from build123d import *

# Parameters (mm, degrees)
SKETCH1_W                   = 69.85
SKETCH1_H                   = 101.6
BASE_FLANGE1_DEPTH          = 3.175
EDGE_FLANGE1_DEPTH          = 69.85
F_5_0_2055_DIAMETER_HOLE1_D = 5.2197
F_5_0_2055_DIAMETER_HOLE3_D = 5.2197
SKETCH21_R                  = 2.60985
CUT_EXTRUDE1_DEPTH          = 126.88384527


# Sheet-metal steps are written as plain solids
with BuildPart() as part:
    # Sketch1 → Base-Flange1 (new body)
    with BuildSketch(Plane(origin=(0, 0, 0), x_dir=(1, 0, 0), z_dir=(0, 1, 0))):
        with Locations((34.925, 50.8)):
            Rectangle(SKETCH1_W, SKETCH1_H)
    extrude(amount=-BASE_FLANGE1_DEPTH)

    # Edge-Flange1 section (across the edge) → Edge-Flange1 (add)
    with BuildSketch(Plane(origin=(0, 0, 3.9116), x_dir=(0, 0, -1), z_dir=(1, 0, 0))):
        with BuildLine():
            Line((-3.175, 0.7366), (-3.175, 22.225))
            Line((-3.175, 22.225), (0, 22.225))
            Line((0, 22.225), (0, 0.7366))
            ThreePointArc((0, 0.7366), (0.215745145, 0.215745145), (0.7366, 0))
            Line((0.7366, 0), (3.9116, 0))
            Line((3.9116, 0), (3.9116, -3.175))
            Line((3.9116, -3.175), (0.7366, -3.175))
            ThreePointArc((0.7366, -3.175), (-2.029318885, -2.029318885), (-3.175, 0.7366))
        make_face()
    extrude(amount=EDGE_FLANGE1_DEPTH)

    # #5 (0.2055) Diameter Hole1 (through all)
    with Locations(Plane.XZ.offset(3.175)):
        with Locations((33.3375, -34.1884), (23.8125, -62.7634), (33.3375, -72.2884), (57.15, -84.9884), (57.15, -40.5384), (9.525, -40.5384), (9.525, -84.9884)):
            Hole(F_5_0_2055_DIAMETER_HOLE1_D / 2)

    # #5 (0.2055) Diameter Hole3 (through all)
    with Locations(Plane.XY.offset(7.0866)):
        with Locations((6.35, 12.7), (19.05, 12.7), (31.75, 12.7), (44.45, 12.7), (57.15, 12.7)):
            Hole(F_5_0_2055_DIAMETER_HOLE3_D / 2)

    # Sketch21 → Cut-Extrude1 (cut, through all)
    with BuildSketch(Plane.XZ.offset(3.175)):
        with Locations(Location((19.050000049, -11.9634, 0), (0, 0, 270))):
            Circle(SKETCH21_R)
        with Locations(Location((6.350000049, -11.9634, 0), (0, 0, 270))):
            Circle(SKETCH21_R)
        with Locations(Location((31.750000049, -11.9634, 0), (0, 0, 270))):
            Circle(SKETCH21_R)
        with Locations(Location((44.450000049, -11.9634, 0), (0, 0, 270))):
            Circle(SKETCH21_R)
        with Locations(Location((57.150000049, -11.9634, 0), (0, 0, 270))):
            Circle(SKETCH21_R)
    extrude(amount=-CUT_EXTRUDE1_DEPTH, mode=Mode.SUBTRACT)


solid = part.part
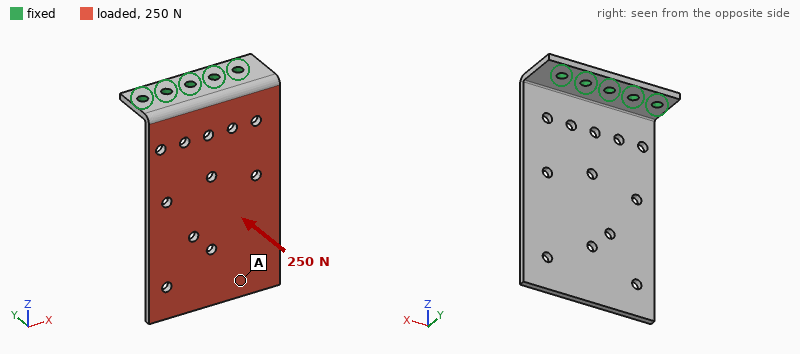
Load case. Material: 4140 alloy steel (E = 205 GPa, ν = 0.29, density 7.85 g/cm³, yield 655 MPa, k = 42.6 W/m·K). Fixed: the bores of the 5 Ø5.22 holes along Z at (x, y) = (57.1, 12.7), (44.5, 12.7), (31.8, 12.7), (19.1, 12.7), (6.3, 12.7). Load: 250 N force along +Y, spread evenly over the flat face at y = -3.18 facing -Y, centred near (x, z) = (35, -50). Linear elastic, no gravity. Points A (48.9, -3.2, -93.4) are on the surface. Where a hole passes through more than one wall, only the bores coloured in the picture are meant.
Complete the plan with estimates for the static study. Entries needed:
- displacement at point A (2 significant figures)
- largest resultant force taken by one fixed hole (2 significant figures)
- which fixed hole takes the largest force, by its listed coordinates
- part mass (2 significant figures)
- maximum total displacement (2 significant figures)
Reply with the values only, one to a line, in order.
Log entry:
1.4 mm
83 N
(19.1, 12.7)
220 g
1.5 mm
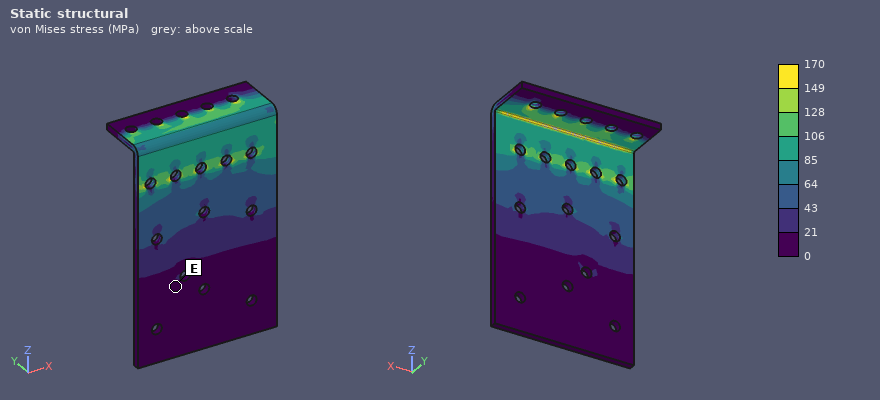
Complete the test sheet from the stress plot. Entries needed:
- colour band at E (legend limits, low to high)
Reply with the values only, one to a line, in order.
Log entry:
0 to 21 MPa
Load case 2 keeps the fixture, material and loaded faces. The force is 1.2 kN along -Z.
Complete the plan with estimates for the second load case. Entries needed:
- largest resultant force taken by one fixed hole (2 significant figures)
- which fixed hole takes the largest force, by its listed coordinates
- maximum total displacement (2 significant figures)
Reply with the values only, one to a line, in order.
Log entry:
320 N
(57.1, 12.7)
0.54 mm
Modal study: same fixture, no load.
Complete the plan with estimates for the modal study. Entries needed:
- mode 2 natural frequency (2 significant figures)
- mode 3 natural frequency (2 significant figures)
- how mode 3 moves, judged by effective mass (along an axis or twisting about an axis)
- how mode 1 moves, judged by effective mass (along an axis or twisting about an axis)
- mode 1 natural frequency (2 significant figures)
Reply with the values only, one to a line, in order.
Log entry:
710 Hz
1100 Hz
along X
along Y
190 Hz
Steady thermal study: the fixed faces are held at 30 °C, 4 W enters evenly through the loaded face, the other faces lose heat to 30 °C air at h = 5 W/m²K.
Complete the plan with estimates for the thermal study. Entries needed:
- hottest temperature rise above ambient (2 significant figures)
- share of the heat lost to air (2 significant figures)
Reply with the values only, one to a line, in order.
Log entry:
24 K
20 %
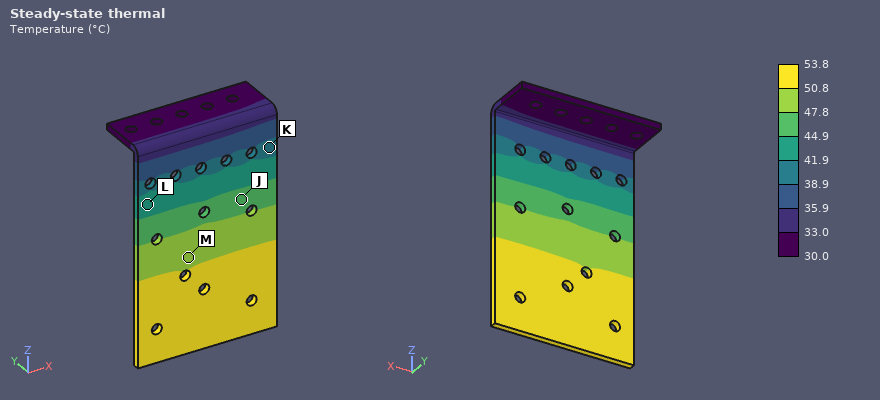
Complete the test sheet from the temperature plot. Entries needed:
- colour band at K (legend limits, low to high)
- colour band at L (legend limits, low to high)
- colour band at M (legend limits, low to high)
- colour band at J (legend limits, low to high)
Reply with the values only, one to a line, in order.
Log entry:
38.9 to 41.9 °C
41.9 to 44.9 °C
47.8 to 50.8 °C
44.9 to 47.8 °C
